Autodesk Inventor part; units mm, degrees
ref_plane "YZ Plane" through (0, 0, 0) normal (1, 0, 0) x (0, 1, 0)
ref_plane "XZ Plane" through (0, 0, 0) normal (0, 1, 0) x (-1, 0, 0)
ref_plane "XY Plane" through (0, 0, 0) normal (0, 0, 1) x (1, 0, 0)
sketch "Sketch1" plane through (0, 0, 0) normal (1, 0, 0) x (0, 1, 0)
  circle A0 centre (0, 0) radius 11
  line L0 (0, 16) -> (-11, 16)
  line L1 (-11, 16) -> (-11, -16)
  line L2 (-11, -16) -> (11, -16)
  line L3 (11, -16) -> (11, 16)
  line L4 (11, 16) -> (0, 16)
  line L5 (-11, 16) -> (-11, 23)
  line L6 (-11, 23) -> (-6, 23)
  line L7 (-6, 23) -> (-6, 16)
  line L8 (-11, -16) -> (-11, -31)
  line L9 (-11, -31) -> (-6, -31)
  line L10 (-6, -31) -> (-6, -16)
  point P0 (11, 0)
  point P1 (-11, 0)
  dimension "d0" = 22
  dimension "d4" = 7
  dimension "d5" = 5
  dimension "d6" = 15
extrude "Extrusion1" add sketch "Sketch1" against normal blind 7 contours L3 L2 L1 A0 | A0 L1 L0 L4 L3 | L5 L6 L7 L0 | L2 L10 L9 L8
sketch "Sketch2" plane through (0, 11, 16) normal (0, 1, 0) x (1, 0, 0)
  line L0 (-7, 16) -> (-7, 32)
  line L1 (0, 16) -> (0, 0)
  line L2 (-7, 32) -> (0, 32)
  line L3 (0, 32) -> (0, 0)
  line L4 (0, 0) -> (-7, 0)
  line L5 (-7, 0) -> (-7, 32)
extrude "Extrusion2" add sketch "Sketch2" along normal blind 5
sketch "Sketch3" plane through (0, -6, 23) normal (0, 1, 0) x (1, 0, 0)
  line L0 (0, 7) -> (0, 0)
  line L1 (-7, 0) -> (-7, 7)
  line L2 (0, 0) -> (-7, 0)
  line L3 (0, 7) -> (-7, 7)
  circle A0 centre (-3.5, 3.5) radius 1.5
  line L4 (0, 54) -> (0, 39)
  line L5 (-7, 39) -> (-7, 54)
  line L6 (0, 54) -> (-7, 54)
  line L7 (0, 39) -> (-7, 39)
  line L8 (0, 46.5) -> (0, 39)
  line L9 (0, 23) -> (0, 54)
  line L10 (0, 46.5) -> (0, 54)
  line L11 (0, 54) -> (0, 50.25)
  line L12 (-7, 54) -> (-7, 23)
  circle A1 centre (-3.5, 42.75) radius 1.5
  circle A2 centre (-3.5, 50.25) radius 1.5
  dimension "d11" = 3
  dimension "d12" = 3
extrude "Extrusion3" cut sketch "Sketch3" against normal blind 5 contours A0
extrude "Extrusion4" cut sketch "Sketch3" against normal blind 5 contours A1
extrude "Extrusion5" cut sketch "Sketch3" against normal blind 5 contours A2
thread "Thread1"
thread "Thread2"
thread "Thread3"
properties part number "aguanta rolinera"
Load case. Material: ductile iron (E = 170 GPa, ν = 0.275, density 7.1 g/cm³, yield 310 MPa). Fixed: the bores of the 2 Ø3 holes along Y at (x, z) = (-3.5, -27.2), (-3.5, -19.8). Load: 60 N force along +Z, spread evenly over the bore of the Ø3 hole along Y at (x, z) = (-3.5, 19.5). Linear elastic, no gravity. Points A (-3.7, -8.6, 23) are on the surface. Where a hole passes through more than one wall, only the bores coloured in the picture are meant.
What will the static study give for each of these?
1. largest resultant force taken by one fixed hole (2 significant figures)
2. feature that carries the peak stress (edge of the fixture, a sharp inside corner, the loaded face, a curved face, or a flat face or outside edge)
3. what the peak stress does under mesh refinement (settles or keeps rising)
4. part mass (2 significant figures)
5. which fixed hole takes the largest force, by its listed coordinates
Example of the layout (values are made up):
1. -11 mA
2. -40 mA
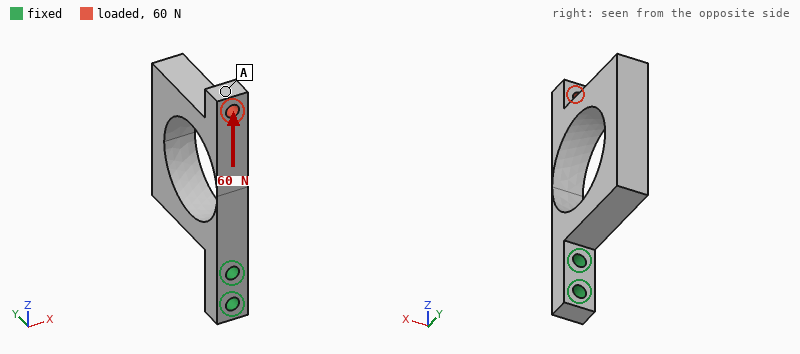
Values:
1. 56 N
2. a sharp inside corner
3. keeps rising
4. 29 g
5. (-3.5, -19.8)
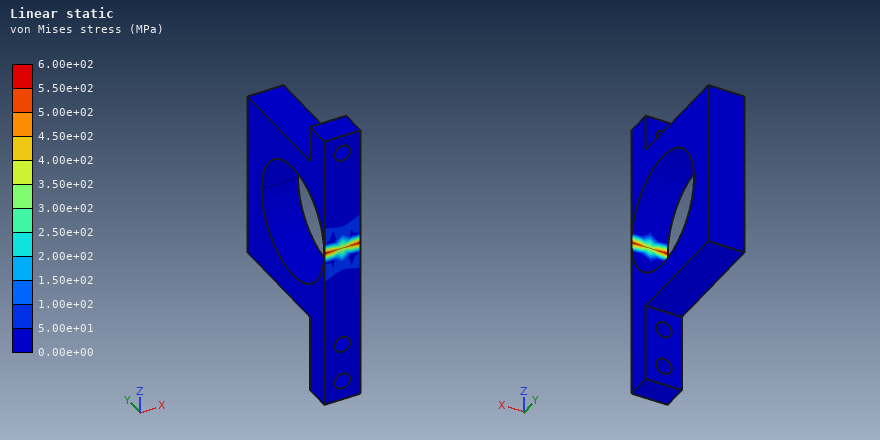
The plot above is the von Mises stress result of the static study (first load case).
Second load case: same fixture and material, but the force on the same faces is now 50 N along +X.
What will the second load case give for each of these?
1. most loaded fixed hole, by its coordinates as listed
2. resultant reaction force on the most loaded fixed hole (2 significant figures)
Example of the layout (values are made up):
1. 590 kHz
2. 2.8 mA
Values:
1. (-3.5, -19.8)
2. 120 N
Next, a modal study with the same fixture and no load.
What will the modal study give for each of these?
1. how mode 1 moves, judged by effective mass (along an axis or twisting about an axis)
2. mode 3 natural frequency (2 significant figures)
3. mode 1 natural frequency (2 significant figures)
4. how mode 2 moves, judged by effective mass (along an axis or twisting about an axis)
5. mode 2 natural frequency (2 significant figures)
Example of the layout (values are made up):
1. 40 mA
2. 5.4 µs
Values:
1. along Y
2. 3000 Hz
3. 1300 Hz
4. along X
5. 1400 Hz
